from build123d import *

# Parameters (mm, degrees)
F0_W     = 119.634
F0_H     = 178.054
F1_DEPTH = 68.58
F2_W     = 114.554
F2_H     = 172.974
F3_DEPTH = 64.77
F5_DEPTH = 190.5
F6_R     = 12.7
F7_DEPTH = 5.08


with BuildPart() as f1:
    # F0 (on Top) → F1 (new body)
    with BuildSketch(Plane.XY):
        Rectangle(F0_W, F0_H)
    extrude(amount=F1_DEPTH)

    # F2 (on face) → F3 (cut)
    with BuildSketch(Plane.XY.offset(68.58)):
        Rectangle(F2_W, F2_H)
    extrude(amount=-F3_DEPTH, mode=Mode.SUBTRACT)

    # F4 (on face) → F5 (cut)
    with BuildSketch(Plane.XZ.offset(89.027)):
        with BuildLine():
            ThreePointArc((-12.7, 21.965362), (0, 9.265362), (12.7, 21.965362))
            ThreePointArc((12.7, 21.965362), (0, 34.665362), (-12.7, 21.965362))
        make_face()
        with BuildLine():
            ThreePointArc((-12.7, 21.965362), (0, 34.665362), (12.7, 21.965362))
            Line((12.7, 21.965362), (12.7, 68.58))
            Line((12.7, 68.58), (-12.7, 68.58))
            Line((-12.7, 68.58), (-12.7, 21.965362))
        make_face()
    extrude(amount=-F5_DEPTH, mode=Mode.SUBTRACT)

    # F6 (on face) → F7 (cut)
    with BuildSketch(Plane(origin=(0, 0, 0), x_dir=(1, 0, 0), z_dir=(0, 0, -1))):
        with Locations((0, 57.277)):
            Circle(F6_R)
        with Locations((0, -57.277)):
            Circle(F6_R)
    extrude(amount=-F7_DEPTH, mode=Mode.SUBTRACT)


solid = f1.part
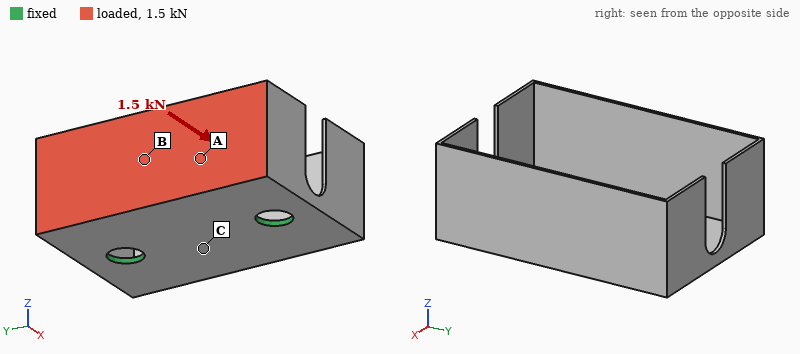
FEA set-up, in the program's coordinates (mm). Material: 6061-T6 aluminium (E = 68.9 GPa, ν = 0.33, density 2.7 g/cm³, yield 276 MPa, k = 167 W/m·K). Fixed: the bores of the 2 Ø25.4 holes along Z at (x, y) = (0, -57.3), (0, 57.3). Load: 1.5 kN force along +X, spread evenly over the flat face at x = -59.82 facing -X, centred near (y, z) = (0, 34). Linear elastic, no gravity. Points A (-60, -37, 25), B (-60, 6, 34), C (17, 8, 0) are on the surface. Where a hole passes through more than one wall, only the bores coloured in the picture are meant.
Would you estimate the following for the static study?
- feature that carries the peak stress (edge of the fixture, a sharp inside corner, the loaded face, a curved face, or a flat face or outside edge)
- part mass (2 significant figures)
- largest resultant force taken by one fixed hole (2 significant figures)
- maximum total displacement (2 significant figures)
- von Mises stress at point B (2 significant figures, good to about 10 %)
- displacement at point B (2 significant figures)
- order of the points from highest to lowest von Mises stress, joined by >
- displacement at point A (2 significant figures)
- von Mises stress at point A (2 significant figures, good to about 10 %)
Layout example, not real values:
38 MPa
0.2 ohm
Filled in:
a curved face
450 g
970 N
2.6 mm
27 MPa
1.2 mm
A > B > C
0.74 mm
51 MPa
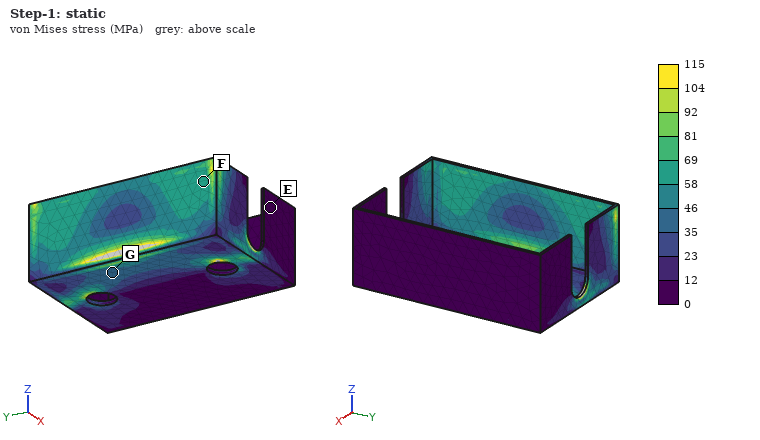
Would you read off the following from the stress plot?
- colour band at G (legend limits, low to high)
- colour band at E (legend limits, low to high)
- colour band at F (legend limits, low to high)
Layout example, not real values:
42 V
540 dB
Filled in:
35 to 46 MPa
0 to 12 MPa
58 to 69 MPa
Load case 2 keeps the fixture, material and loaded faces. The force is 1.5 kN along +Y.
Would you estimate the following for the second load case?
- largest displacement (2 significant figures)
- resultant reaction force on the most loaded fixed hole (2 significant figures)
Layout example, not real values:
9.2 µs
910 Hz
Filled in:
0.62 mm
1.0 kN
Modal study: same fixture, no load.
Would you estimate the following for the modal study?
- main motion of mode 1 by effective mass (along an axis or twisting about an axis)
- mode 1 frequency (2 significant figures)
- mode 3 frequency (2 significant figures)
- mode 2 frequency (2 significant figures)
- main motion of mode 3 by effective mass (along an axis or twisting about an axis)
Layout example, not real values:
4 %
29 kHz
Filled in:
along X
450 Hz
540 Hz
500 Hz
along Z
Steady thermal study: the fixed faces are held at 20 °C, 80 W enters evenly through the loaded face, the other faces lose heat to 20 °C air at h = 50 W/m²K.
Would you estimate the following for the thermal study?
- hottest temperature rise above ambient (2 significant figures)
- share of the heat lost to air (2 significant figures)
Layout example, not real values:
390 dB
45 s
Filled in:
39 K
53 %
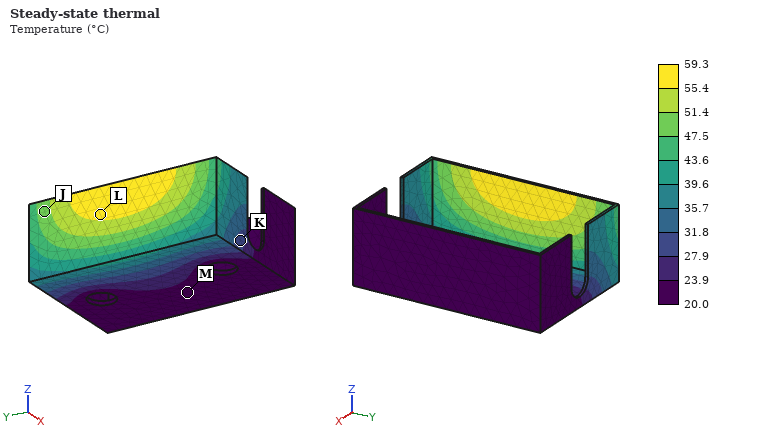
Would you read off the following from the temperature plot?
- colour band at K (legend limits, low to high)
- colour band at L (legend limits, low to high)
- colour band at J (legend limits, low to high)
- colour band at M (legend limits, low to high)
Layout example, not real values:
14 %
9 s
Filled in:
27.9 to 31.8 °C
55.4 to 59.3 °C
47.5 to 51.4 °C
20.0 to 23.9 °C
